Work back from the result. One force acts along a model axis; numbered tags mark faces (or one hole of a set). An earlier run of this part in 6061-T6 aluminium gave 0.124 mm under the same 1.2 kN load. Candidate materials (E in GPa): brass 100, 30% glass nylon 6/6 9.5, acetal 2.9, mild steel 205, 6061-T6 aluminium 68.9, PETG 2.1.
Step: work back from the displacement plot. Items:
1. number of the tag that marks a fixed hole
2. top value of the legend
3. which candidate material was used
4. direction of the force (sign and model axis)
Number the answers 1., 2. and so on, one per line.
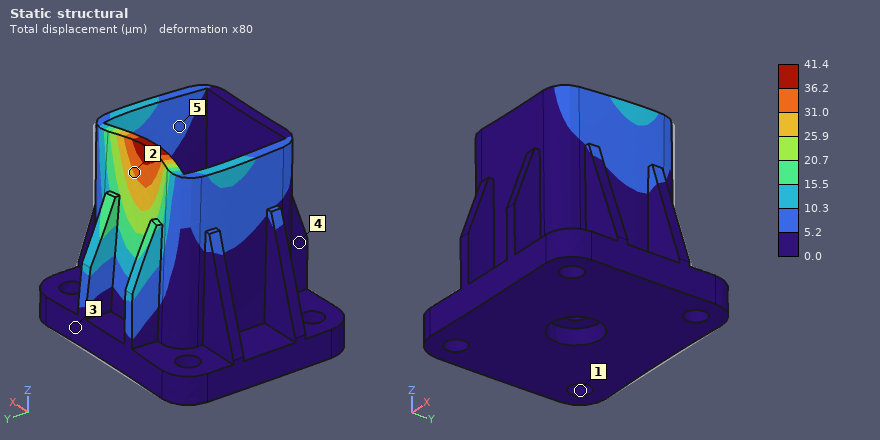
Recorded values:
1. 1
2. 41.4 µm
3. mild steel
4. -Y
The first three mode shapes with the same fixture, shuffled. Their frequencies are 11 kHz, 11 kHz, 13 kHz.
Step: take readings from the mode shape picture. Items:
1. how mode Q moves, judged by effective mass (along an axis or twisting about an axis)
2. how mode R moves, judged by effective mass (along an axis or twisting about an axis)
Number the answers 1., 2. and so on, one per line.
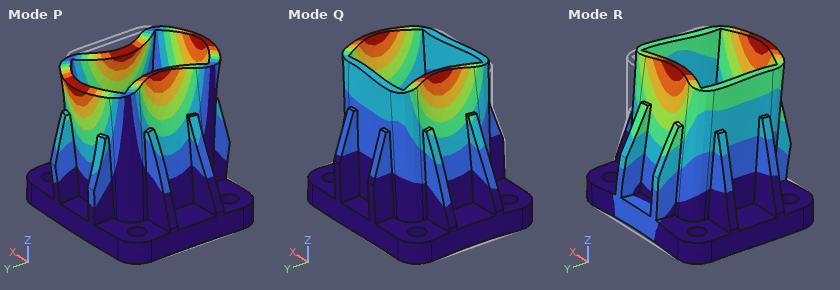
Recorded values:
1. along X
2. along Y
